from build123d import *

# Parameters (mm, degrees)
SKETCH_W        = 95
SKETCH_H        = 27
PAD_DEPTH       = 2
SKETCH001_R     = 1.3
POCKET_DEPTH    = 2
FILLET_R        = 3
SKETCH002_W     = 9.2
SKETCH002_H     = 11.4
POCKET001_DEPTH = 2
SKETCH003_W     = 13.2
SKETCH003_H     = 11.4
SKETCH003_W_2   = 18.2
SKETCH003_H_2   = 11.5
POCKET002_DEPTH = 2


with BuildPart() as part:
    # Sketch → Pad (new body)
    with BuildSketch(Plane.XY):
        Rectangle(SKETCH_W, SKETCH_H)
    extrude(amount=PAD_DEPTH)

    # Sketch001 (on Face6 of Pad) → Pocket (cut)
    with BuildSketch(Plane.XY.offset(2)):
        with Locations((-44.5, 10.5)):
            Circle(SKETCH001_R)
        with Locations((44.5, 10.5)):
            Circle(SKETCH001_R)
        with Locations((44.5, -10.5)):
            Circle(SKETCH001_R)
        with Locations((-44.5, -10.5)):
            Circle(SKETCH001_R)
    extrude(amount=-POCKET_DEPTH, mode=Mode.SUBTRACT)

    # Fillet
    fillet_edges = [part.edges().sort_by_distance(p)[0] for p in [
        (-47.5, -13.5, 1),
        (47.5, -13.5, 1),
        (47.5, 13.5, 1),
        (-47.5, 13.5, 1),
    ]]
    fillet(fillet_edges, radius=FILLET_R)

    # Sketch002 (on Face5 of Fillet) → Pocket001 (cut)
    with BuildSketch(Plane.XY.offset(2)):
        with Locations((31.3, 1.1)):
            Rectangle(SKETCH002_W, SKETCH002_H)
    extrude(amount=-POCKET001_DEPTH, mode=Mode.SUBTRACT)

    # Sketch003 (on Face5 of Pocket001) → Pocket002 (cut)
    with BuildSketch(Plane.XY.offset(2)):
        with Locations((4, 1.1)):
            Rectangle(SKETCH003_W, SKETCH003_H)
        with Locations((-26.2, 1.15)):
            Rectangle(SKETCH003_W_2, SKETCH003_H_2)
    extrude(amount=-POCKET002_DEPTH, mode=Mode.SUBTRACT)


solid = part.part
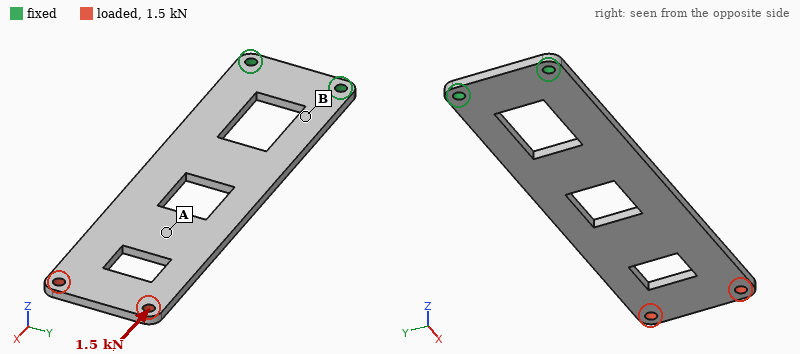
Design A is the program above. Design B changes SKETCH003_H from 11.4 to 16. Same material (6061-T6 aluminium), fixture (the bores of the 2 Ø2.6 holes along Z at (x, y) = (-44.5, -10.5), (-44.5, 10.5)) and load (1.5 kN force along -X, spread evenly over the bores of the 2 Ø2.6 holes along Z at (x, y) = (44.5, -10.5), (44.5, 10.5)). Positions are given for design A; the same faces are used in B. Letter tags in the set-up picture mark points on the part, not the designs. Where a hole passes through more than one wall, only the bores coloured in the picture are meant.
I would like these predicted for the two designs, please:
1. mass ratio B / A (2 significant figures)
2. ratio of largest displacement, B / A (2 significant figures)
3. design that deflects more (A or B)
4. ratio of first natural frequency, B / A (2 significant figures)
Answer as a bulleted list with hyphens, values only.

- 0.97
- 1.2
- B
- 0.99
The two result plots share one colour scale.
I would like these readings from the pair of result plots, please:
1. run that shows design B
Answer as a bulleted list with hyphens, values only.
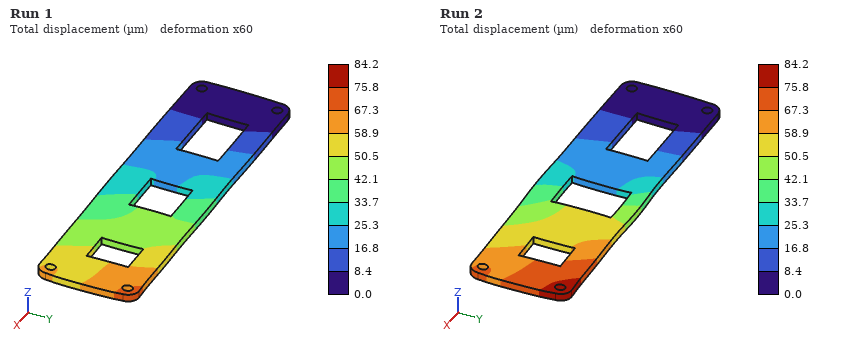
- Run 2
